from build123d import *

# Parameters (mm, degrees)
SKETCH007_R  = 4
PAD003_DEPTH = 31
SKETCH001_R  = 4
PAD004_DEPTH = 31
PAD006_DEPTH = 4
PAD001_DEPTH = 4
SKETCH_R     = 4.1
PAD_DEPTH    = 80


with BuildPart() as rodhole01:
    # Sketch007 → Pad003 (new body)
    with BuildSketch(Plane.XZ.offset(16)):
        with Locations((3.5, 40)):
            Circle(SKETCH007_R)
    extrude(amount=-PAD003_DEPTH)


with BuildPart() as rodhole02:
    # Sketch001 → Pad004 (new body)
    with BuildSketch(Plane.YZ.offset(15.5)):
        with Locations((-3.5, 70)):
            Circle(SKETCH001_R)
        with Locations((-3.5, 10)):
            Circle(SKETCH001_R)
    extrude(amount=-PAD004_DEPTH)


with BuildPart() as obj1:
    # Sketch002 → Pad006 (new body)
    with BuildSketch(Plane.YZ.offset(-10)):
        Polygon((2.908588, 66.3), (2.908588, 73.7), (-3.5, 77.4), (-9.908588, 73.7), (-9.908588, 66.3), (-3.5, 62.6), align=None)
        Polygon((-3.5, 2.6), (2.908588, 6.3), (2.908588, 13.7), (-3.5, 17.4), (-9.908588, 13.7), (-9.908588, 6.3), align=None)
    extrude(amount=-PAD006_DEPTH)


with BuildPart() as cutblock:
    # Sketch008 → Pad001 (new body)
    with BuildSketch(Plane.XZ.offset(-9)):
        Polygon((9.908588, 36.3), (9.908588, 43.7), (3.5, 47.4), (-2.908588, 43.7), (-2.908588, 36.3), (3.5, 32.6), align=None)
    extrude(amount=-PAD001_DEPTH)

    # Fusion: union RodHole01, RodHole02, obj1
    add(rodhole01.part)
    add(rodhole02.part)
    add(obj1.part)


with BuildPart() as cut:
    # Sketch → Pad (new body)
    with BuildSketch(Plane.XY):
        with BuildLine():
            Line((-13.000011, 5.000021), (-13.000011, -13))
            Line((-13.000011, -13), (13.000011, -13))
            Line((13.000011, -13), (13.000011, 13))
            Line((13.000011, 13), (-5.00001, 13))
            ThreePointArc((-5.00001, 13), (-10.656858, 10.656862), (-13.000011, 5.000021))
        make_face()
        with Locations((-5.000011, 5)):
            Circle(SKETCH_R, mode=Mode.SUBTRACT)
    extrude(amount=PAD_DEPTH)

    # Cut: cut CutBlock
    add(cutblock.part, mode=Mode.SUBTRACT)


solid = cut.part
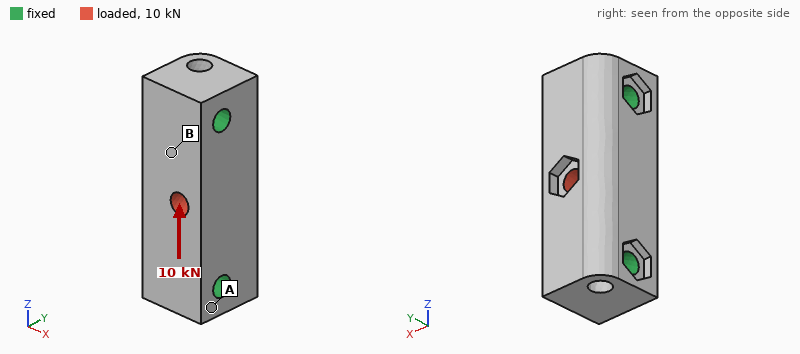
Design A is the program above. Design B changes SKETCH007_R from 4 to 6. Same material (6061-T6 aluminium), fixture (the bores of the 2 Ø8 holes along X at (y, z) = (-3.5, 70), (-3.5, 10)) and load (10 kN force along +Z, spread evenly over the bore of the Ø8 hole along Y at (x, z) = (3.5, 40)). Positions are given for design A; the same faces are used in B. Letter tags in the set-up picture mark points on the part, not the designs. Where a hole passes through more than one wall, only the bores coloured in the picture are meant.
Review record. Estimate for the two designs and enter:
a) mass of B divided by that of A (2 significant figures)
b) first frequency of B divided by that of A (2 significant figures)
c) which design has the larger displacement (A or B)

0.97
1.0
A
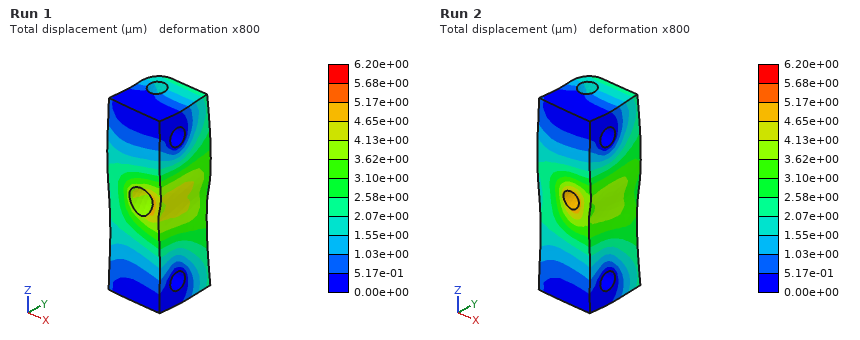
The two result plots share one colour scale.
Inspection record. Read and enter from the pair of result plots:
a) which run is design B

Run 1
